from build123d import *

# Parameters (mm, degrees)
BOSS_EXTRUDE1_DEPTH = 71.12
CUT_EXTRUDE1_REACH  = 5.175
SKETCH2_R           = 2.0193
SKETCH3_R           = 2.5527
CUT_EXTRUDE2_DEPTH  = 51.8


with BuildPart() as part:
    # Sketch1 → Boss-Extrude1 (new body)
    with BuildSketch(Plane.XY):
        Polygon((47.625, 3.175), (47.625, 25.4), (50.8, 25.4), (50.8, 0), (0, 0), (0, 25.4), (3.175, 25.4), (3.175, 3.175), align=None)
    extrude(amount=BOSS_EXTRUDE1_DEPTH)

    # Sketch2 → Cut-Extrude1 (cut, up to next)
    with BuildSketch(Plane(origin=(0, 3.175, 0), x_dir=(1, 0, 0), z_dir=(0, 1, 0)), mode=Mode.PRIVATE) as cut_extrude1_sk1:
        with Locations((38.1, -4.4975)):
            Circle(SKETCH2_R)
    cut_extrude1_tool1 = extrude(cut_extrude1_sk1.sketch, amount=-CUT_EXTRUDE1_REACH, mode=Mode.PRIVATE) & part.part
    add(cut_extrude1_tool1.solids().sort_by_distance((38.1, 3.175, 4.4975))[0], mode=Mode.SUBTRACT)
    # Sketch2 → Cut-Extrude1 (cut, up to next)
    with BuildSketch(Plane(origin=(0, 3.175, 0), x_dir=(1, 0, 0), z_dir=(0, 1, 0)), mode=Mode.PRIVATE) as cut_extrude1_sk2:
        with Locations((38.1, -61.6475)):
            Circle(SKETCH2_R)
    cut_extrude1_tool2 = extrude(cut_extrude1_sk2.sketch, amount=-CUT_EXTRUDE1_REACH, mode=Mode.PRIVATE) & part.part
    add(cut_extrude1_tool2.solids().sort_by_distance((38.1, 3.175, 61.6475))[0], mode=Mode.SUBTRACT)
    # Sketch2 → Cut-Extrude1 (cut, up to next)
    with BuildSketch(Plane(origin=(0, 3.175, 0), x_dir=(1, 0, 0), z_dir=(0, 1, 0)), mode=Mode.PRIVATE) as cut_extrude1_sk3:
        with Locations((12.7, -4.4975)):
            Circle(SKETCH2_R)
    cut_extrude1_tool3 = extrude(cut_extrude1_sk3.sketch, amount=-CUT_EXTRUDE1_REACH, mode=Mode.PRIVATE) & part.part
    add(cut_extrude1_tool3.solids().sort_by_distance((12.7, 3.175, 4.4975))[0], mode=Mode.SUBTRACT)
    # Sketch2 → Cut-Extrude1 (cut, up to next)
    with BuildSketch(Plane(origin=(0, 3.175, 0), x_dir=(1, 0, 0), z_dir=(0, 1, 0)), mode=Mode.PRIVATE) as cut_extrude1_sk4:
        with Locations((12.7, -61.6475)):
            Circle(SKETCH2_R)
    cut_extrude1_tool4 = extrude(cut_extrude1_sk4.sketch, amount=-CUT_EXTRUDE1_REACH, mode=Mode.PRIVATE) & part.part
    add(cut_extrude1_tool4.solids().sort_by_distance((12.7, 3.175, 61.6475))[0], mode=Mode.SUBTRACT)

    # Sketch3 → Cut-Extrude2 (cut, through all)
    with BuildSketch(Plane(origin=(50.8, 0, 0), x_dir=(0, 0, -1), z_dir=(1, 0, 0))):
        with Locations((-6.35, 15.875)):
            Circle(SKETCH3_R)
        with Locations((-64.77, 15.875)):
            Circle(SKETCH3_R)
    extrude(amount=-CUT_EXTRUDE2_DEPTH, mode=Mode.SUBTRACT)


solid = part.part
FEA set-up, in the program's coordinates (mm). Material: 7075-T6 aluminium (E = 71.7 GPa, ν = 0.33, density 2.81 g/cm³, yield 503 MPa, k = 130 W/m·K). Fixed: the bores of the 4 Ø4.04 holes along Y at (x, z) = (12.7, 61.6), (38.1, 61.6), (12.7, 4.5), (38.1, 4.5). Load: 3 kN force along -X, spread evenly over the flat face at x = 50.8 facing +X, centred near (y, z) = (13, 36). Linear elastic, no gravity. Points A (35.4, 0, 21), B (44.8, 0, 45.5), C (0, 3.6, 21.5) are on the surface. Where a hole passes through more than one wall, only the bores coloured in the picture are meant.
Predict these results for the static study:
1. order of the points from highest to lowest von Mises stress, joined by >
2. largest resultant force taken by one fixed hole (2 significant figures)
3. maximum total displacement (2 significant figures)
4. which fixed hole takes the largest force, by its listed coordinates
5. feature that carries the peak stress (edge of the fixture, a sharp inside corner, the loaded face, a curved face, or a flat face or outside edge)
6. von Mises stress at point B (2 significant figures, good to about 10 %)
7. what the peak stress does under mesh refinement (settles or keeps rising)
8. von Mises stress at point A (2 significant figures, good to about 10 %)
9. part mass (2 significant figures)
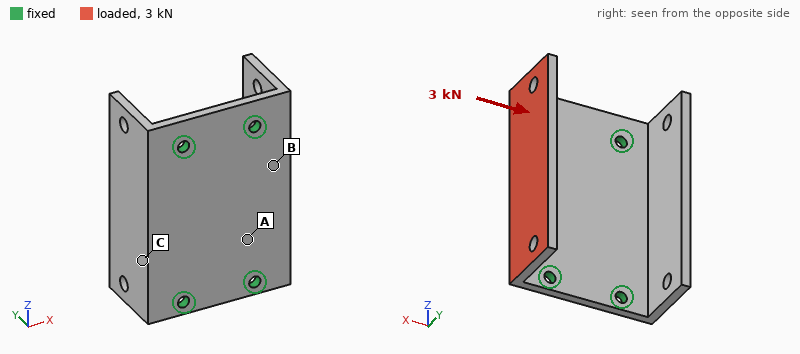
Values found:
B > A > C
1.1 kN
1.0 mm
(38.1, 61.6)
edge of the fixture
200 MPa
keeps rising
110 MPa
59 g
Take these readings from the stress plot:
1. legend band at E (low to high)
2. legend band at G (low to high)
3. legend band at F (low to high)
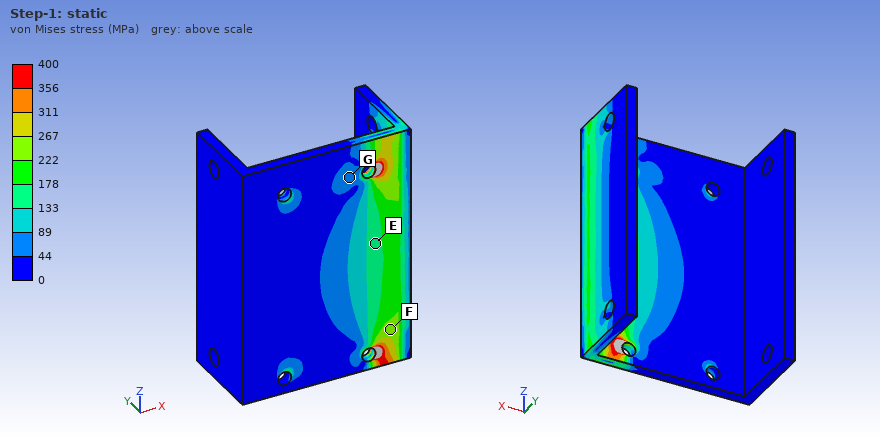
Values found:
133 to 178 MPa
44 to 89 MPa
222 to 267 MPa
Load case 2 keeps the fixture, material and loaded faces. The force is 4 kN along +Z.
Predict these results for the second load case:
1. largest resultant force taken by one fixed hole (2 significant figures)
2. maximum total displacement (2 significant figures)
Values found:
2.2 kN
0.12 mm
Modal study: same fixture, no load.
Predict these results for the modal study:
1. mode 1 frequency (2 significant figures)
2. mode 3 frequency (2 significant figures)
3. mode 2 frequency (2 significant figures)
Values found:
2500 Hz
4100 Hz
2600 Hz
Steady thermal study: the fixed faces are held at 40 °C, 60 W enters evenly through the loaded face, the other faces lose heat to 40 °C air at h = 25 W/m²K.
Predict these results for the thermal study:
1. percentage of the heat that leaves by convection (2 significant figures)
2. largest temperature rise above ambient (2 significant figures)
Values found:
8.1 %
56 K
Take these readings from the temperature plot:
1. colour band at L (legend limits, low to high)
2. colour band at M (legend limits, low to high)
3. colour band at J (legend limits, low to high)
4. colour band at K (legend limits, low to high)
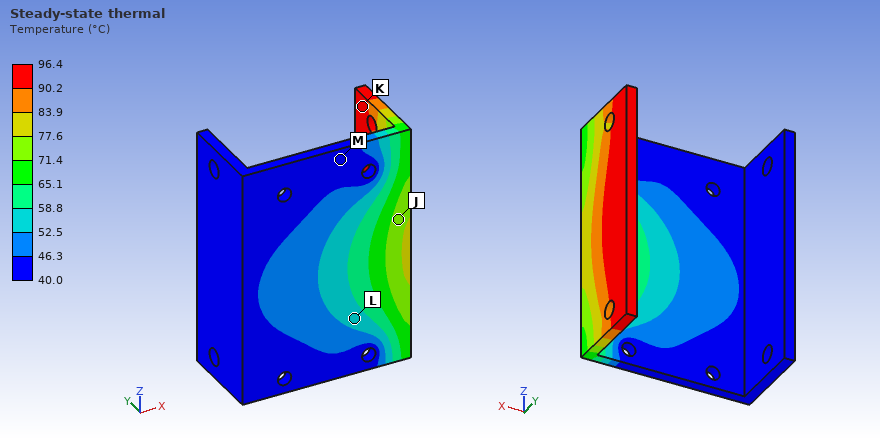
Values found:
52.5 to 58.8 °C
40.0 to 46.3 °C
71.4 to 77.6 °C
90.2 to 96.4 °C
